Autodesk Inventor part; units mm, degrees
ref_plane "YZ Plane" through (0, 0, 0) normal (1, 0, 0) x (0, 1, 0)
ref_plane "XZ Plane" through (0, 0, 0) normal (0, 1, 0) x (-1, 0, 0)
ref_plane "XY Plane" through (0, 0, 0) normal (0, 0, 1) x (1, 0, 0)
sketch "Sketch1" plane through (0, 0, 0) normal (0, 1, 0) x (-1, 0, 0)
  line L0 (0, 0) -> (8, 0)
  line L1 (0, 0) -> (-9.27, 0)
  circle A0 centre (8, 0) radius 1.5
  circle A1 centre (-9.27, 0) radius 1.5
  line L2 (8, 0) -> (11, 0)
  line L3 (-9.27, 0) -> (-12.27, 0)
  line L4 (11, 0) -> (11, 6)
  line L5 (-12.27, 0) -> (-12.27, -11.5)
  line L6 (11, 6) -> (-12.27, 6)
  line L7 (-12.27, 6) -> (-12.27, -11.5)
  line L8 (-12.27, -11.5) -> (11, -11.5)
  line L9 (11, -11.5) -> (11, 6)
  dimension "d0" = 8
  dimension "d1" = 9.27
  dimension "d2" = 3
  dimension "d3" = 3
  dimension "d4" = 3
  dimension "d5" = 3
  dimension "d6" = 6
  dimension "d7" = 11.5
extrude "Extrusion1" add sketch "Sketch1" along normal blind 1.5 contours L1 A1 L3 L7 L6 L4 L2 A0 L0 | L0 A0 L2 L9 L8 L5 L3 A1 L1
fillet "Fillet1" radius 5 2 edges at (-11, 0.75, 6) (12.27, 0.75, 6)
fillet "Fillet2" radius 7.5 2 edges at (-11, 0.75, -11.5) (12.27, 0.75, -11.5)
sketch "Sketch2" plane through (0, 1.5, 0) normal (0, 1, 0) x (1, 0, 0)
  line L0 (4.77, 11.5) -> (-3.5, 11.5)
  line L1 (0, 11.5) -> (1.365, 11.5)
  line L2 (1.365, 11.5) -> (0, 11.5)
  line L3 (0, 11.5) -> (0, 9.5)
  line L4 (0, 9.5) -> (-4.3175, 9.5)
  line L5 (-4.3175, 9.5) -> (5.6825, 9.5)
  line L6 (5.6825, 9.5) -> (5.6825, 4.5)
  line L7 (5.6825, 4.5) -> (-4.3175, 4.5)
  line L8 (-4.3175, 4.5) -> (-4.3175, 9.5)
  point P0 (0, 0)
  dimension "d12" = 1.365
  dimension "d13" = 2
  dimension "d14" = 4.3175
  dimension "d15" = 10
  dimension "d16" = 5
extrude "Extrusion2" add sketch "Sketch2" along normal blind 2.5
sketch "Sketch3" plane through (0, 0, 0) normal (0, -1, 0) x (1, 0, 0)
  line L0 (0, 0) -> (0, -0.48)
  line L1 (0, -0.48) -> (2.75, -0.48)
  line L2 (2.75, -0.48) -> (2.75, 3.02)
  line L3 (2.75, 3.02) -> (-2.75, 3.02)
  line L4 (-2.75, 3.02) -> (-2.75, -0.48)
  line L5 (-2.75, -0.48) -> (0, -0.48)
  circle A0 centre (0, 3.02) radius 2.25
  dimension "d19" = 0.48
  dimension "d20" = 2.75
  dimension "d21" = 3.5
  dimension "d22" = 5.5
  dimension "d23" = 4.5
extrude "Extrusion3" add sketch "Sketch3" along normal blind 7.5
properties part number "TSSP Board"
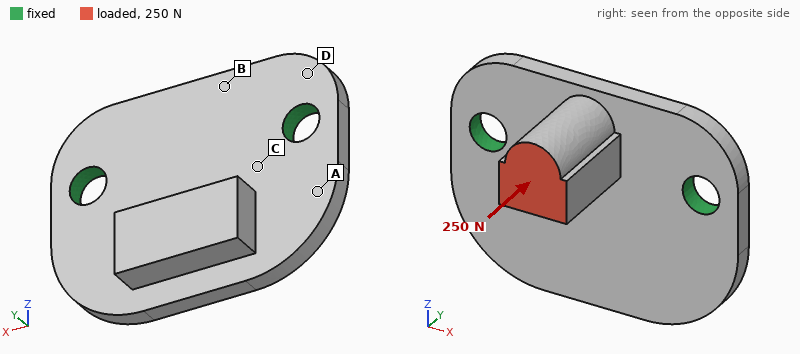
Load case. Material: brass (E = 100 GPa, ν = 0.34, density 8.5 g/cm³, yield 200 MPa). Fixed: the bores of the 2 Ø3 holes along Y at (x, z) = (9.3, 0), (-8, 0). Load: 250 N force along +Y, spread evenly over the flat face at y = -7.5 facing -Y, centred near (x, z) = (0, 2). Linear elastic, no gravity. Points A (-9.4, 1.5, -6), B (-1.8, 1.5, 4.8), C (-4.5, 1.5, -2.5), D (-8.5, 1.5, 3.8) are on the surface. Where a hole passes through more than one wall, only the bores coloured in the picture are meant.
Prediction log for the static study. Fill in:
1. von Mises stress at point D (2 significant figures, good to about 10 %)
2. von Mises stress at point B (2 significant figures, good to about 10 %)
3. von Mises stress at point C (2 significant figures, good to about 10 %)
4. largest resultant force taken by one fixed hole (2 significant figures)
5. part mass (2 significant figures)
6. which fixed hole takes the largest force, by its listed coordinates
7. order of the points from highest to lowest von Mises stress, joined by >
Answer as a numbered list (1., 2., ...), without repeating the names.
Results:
1. 52 MPa
2. 65 MPa
3. 34 MPa
4. 140 N
5. 7.4 g
6. (-8, 0)
7. B > D > C > A
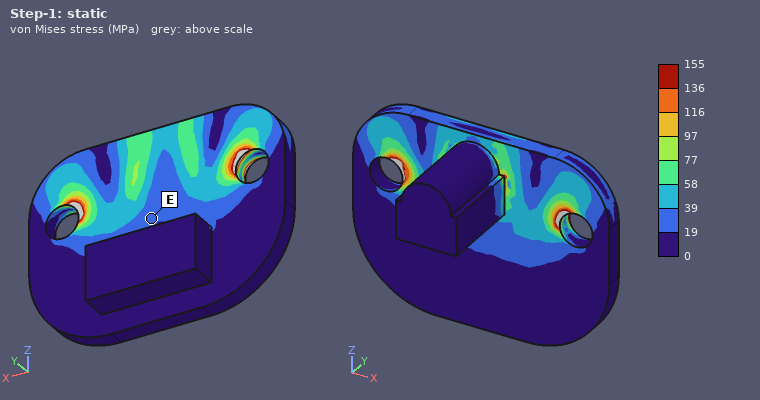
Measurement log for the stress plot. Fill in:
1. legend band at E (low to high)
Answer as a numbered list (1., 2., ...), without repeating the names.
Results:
1. 19 to 39 MPa
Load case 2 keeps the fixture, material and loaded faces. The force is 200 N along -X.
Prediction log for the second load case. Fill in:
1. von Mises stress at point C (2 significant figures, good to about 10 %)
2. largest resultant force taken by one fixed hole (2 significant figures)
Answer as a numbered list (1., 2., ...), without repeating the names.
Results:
1. 28 MPa
2. 180 N
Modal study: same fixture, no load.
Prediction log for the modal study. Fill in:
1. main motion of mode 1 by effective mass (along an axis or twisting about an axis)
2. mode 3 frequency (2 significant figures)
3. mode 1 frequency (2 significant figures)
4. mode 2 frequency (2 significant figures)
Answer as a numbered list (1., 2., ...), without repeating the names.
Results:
1. along Y
2. 15 kHz
3. 5900 Hz
4. 9200 Hz
